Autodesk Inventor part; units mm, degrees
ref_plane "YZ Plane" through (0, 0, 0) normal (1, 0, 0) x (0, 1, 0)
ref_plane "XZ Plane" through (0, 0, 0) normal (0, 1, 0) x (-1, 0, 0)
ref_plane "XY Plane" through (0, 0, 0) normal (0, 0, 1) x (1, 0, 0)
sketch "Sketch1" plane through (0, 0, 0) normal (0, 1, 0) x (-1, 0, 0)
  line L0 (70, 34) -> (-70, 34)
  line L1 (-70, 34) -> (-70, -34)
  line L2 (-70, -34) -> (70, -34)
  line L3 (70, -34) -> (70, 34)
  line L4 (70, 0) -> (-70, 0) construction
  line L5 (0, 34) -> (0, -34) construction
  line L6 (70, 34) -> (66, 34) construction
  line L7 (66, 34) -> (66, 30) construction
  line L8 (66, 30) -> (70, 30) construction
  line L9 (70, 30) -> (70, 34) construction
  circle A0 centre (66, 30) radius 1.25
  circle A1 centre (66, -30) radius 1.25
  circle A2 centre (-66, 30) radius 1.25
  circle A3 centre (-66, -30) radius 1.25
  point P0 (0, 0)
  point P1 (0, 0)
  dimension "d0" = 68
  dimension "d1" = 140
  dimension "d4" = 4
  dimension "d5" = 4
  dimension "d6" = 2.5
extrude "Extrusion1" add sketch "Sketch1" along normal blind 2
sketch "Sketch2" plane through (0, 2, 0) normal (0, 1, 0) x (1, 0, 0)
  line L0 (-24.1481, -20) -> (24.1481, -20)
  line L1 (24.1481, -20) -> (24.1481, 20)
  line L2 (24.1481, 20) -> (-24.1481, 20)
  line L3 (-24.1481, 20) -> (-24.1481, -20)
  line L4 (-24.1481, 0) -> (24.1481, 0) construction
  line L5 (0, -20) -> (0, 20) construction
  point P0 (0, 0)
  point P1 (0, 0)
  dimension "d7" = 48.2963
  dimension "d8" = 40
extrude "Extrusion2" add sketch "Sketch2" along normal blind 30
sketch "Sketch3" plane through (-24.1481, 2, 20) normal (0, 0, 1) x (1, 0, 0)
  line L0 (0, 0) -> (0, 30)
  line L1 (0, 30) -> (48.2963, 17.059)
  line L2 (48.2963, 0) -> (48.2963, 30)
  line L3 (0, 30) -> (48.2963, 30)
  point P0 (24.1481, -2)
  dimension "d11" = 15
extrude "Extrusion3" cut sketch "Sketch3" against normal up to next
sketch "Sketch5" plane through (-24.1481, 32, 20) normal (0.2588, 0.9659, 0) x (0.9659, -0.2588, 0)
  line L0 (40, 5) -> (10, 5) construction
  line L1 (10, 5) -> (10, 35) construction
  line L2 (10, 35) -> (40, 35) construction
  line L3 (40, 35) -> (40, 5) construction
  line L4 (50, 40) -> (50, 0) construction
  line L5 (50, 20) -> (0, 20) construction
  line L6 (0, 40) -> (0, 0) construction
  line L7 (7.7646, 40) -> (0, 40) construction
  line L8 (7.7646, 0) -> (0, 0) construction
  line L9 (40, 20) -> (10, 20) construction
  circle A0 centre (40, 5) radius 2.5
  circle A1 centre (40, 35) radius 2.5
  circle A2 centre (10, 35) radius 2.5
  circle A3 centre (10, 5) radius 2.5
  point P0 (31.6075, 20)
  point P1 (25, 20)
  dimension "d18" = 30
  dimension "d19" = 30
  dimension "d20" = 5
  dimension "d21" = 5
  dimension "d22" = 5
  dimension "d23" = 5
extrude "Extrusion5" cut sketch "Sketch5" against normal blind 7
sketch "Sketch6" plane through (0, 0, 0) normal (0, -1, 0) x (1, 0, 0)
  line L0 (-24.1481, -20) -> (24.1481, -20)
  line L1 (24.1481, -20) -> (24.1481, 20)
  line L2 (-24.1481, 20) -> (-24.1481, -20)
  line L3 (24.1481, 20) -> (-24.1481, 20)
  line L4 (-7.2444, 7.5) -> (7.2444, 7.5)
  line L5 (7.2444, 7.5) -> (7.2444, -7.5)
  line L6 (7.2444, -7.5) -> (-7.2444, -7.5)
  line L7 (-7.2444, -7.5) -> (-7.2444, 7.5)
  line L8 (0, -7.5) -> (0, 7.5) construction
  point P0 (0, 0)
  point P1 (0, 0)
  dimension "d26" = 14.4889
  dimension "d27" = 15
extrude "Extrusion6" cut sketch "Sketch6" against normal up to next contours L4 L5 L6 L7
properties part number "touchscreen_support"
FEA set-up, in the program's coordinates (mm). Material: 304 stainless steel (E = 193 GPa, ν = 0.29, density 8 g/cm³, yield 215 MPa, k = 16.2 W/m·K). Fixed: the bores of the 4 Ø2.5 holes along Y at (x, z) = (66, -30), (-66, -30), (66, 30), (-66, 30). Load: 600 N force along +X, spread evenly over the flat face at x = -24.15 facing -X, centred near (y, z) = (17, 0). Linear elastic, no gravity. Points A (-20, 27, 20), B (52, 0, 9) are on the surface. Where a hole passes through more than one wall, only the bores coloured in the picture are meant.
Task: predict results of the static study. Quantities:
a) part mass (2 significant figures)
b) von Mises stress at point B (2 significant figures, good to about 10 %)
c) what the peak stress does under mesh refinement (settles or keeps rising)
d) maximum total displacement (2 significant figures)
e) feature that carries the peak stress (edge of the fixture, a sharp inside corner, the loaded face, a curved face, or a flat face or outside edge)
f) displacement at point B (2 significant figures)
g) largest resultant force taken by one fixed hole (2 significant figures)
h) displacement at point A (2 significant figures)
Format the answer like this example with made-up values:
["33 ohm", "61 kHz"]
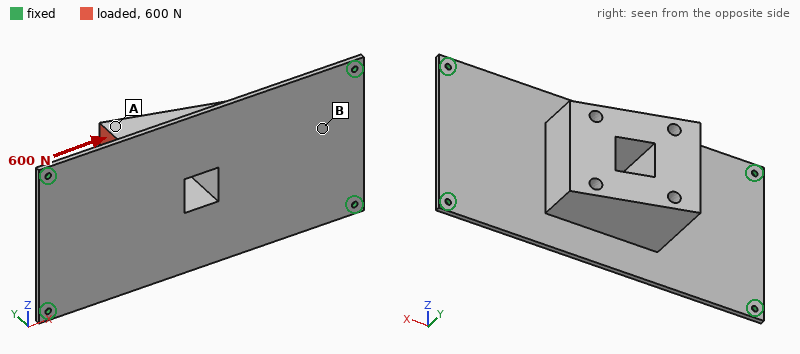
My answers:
["470 g", "8.9 MPa", "keeps rising", "86 µm", "edge of the fixture", "36 µm", "170 N", "72 µm"]
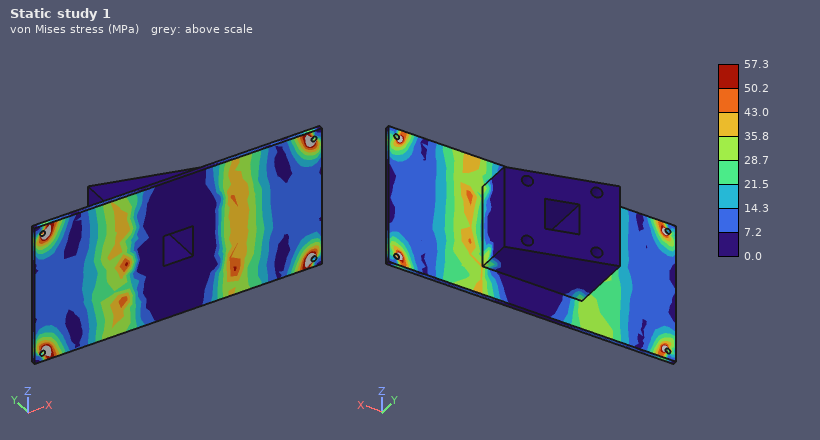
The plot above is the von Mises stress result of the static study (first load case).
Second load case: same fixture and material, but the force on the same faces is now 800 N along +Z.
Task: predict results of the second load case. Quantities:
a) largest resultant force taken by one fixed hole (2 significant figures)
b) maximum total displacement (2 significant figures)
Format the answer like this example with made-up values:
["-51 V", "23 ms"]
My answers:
["360 N", "0.32 mm"]
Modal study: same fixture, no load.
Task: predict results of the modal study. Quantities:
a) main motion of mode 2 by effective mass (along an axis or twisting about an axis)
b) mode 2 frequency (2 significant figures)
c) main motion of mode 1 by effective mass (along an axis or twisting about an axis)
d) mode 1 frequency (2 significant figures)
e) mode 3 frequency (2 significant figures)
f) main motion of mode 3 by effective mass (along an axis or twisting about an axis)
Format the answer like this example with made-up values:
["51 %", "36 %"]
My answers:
["along Z", "500 Hz", "along Y", "330 Hz", "780 Hz", "along X"]
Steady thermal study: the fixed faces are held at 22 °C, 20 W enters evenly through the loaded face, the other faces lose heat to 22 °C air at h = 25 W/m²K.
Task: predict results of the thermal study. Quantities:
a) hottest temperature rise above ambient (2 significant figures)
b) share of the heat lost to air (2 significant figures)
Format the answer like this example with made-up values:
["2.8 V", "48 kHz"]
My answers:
["76 K", "93 %"]
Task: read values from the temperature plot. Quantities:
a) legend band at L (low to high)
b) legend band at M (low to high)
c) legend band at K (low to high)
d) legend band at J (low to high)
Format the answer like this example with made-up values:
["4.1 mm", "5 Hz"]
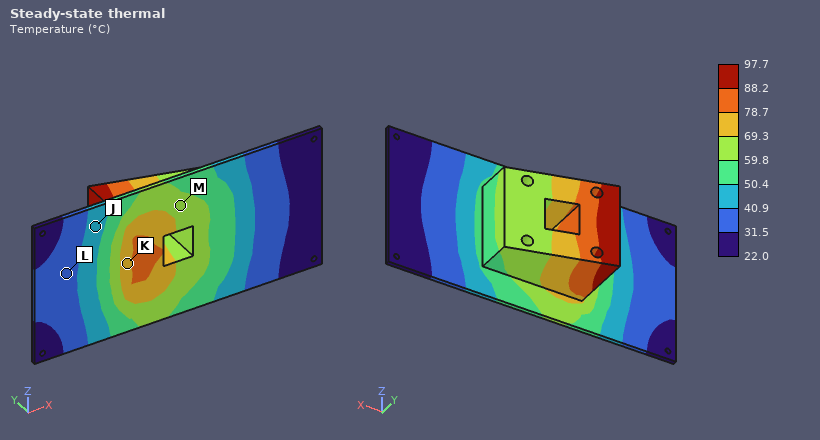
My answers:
["31.5 to 40.9 °C", "59.8 to 69.3 °C", "69.3 to 78.7 °C", "40.9 to 50.4 °C"]
